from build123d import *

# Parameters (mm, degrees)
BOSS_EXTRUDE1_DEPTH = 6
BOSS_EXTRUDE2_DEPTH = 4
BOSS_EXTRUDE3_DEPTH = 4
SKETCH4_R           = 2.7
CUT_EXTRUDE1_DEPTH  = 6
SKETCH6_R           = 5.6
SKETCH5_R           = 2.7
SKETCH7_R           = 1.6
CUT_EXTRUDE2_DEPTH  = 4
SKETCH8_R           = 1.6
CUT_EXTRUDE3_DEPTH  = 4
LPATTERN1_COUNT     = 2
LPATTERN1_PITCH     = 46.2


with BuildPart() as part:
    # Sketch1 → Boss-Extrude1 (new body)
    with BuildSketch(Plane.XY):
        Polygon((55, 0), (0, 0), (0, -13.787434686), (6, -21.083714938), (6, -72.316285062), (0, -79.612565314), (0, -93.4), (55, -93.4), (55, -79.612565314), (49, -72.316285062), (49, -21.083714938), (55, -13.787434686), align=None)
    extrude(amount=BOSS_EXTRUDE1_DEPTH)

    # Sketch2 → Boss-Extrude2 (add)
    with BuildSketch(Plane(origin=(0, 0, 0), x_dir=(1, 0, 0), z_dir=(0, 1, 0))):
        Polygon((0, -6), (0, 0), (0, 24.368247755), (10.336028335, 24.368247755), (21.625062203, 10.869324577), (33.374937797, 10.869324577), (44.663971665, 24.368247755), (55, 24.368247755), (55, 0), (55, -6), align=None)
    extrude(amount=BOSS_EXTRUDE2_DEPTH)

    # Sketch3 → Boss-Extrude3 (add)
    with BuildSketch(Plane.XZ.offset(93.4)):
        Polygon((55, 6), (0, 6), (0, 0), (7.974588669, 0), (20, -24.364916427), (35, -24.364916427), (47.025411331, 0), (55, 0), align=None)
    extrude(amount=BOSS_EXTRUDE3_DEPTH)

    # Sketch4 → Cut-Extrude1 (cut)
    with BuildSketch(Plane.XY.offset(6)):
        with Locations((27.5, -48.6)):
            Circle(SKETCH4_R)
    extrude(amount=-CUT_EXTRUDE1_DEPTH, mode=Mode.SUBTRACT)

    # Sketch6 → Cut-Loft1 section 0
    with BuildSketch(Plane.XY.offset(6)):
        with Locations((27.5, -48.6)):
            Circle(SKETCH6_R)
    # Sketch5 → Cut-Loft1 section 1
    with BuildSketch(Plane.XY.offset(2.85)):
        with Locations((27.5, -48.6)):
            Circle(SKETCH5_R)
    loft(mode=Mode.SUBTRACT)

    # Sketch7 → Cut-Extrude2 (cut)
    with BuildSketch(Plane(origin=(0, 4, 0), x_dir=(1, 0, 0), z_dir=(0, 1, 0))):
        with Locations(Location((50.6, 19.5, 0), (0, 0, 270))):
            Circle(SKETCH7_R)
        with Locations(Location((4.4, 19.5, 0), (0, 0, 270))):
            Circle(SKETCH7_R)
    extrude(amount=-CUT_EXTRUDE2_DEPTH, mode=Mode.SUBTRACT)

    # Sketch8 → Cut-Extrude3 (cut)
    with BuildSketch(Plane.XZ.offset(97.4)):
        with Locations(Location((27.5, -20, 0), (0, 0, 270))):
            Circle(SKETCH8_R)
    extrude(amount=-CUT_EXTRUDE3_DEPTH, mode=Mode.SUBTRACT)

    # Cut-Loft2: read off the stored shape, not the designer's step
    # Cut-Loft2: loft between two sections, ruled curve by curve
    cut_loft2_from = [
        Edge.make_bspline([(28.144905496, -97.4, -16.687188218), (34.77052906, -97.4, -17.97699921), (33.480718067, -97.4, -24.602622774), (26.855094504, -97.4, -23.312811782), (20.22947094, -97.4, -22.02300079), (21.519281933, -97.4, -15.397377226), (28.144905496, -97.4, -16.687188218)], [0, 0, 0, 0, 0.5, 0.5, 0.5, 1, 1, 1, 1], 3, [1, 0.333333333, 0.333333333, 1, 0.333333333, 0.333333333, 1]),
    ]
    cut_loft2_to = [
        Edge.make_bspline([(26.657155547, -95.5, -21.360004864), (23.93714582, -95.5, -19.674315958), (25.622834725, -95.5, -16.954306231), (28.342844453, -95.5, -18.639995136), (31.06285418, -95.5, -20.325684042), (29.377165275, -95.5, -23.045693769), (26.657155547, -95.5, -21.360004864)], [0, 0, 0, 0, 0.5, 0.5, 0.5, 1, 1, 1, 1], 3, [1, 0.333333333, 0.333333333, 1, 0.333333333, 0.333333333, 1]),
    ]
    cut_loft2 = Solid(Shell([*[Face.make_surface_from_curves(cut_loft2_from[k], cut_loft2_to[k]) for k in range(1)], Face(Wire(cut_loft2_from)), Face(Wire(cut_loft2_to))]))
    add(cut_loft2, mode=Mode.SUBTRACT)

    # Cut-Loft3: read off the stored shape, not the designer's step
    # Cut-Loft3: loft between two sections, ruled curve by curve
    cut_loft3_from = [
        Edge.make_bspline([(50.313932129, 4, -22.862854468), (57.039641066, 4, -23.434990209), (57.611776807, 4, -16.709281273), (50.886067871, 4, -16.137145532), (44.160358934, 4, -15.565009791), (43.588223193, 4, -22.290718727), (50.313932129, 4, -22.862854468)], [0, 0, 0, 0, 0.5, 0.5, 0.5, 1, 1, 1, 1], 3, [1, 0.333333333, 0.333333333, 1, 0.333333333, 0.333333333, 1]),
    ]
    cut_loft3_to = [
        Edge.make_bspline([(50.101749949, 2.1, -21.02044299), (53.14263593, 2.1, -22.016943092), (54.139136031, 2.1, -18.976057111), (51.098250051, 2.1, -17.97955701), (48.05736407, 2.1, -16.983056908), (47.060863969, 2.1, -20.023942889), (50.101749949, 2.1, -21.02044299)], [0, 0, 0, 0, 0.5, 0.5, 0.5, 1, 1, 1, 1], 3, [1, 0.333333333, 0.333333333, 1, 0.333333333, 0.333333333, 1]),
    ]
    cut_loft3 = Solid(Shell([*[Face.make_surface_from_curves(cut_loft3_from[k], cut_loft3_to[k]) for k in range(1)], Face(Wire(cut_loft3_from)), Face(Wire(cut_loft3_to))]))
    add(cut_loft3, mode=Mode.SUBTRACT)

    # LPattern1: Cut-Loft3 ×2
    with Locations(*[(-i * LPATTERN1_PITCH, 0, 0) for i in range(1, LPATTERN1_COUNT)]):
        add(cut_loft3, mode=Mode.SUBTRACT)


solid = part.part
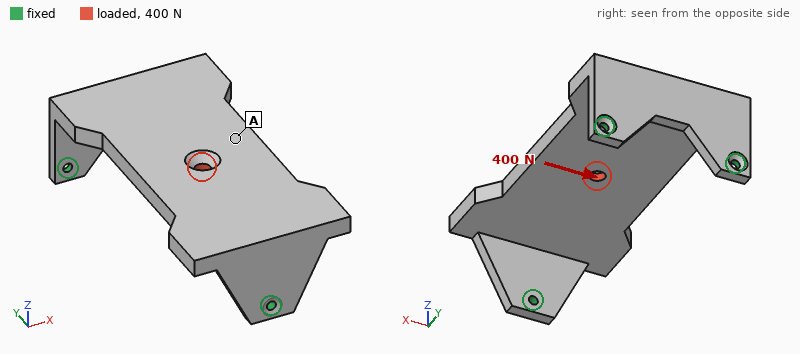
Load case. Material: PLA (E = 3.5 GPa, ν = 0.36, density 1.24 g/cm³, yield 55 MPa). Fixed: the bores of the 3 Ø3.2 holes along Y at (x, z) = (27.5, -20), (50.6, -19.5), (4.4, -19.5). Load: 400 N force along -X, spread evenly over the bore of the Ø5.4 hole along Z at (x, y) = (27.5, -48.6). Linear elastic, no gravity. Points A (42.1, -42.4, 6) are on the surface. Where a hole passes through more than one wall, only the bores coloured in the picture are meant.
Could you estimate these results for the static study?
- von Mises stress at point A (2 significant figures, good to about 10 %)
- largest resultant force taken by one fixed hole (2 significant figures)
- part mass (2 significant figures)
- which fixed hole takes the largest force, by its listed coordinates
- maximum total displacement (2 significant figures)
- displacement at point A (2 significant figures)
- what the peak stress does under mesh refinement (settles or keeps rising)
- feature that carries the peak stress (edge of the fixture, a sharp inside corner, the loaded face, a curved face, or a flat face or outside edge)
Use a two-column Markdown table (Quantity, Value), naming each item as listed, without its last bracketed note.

| Quantity | Value |
|---|---|
| von Mises stress at point A | 5.9 MPa |
| largest resultant force taken by one fixed hole | 190 N |
| part mass | 44 g |
| which fixed hole takes the largest force, by its listed coordinates | (27.5, -20) |
| maximum total displacement | 0.86 mm |
| displacement at point A | 0.38 mm |
| what the peak stress does under mesh refinement | keeps rising |
| feature that carries the peak stress | edge of the fixture |
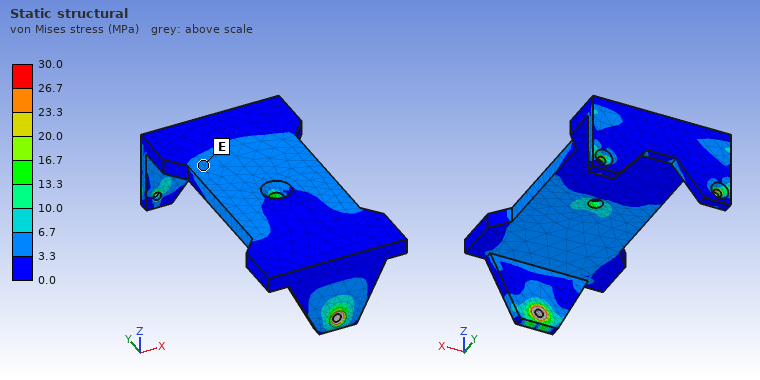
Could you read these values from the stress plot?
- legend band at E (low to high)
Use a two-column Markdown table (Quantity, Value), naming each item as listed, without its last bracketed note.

| Quantity | Value |
|---|---|
| legend band at E | 3.3 to 6.7 MPa |
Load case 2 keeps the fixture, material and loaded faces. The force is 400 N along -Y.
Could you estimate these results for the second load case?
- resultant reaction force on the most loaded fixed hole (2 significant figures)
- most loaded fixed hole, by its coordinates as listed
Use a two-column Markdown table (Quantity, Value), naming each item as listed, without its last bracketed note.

| Quantity | Value |
|---|---|
| resultant reaction force on the most loaded fixed hole | 200 N |
| most loaded fixed hole, by its coordinates as listed | (27.5, -20) |
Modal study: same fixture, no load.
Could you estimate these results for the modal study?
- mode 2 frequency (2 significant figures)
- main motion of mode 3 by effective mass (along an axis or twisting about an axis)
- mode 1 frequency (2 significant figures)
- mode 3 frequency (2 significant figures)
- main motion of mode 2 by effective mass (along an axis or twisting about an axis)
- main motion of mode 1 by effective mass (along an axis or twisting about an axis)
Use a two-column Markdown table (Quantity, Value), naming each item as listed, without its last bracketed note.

| Quantity | Value |
|---|---|
| mode 2 frequency | 670 Hz |
| main motion of mode 3 by effective mass | along Z |
| mode 1 frequency | 640 Hz |
| mode 3 frequency | 720 Hz |
| main motion of mode 2 by effective mass | along X |
| main motion of mode 1 by effective mass | along Y |
